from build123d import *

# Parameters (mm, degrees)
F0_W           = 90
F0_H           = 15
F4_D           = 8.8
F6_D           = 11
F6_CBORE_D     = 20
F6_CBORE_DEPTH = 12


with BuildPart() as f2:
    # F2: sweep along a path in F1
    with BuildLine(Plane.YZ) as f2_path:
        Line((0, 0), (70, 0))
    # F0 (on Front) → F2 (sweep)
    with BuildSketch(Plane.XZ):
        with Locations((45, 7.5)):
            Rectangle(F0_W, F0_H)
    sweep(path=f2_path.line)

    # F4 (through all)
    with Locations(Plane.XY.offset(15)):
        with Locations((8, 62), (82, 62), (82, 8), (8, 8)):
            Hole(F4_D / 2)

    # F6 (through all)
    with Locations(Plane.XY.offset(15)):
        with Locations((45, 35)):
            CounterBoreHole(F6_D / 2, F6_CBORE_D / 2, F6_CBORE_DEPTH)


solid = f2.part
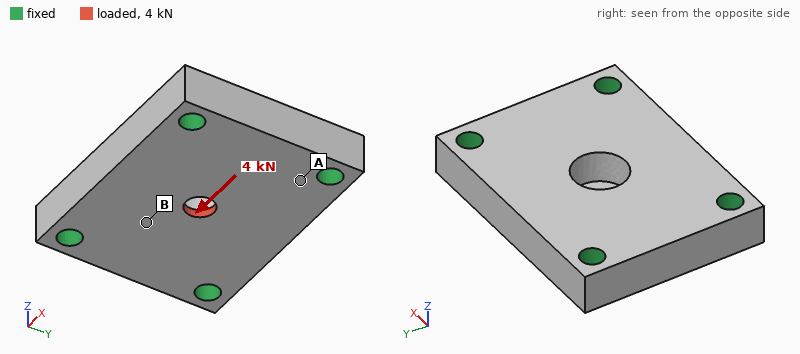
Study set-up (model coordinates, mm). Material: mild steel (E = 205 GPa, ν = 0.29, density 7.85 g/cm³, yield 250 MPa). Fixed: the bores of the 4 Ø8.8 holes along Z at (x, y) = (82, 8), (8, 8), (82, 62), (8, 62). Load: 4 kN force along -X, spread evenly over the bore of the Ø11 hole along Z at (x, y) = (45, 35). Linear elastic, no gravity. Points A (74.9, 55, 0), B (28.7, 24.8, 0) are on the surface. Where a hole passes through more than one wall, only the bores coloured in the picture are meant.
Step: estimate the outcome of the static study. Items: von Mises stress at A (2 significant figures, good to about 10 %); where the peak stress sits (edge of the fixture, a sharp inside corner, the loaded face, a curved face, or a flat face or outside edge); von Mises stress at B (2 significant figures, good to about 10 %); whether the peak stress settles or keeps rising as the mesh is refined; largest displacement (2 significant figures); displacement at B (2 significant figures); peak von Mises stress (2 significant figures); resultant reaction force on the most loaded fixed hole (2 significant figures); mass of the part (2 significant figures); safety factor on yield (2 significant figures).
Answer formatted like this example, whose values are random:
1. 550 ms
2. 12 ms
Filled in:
1. 4.7 MPa
2. the loaded face
3. 9.1 MPa
4. settles
5. 2.5 µm
6. 0.62 µm
7. 69 MPa
8. 1.1 kN
9. 680 g
10. 3.6
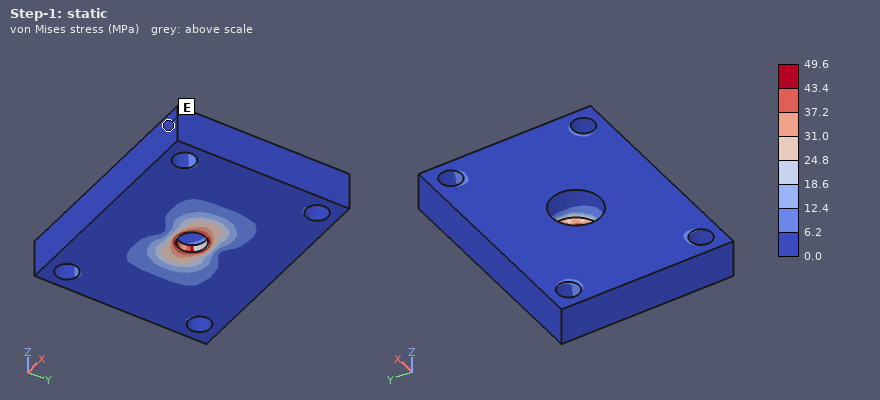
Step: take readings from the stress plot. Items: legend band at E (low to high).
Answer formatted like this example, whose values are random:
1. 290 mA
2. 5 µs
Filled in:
1. 0.0 to 6.2 MPa
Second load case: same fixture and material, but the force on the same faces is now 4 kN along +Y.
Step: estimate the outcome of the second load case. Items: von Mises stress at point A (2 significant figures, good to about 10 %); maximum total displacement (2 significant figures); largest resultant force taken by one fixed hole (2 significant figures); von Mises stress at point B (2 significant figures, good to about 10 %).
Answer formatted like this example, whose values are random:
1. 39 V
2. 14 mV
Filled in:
1. 5.7 MPa
2. 2.9 µm
3. 1.2 kN
4. 8.0 MPa
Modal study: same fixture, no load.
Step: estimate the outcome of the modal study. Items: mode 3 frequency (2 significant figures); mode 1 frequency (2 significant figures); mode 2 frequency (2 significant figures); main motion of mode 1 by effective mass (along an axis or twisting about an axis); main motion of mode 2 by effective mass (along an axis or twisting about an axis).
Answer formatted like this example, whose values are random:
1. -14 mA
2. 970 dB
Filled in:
1. 19 kHz
2. 11 kHz
3. 14 kHz
4. along Z
5. twisting about X
